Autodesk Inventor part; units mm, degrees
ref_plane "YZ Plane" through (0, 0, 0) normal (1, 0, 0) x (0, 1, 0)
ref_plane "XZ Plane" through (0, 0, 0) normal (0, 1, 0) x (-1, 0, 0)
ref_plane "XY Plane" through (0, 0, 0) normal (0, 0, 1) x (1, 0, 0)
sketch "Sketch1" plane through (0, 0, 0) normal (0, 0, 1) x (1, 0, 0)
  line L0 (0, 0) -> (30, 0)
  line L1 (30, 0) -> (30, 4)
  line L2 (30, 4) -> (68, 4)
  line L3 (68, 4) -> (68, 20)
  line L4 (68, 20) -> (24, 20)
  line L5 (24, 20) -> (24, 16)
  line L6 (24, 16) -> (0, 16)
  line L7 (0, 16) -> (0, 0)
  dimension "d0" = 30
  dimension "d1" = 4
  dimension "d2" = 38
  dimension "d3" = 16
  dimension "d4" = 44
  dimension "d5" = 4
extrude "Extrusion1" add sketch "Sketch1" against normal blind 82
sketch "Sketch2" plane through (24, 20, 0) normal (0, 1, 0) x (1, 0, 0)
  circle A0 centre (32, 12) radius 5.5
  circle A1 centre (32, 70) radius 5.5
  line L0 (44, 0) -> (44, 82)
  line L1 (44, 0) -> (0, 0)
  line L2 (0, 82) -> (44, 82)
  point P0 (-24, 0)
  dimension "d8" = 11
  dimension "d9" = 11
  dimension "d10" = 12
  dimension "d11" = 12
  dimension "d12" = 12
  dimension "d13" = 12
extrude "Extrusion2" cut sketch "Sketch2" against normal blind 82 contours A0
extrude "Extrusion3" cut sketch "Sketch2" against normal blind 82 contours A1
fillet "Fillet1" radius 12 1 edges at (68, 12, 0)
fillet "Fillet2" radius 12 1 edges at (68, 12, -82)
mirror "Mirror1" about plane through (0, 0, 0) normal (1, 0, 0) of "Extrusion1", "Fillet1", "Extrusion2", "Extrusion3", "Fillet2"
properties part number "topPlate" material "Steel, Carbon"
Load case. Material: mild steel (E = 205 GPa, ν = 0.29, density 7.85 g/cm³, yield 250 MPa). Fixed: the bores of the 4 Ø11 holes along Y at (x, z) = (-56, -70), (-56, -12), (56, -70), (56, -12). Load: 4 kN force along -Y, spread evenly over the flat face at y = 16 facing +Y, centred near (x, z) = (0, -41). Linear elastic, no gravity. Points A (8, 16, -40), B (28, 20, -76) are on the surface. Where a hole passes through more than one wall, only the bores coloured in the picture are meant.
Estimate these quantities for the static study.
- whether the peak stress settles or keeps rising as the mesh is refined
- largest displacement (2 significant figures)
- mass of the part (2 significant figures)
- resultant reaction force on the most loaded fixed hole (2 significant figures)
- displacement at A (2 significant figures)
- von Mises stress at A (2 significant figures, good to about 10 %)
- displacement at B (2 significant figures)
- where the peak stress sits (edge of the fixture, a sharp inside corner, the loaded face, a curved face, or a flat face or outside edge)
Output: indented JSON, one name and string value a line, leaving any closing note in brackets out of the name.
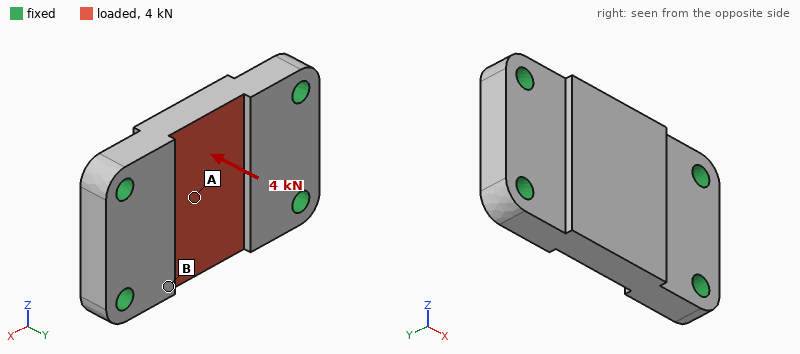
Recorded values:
{
  "whether the peak stress settles or keeps rising as the mesh is refined": "keeps rising",
  "largest displacement": "5.1 µm",
  "mass of the part": "1.4 kg",
  "resultant reaction force on the most loaded fixed hole": "1.3 kN",
  "displacement at A": "4.7 µm",
  "von Mises stress at A": "5.7 MPa",
  "displacement at B": "2.9 µm",
  "where the peak stress sits": "edge of the fixture"
}
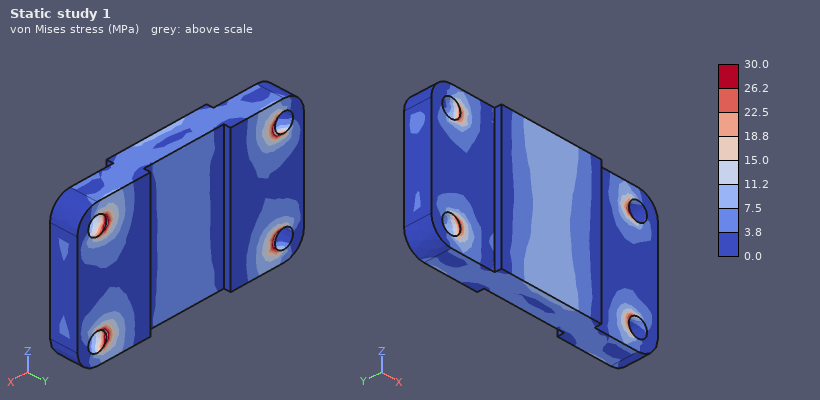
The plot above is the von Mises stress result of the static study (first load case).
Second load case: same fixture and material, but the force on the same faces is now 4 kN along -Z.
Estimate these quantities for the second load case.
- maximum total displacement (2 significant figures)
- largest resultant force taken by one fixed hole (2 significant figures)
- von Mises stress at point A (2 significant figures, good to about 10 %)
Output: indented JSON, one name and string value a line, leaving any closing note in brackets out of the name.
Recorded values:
{
  "maximum total displacement": "1.8 µm",
  "largest resultant force taken by one fixed hole": "1.2 kN",
  "von Mises stress at point A": "2.4 MPa"
}
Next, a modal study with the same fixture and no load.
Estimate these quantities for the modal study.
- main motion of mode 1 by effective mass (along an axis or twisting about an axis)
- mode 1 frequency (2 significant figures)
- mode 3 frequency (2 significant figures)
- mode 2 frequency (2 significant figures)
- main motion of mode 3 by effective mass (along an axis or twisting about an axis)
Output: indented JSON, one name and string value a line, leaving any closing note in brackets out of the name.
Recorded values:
{
  "main motion of mode 1 by effective mass": "along Y",
  "mode 1 frequency": "6000 Hz",
  "mode 3 frequency": "12 kHz",
  "mode 2 frequency": "8200 Hz",
  "main motion of mode 3 by effective mass": "along Z"
}
